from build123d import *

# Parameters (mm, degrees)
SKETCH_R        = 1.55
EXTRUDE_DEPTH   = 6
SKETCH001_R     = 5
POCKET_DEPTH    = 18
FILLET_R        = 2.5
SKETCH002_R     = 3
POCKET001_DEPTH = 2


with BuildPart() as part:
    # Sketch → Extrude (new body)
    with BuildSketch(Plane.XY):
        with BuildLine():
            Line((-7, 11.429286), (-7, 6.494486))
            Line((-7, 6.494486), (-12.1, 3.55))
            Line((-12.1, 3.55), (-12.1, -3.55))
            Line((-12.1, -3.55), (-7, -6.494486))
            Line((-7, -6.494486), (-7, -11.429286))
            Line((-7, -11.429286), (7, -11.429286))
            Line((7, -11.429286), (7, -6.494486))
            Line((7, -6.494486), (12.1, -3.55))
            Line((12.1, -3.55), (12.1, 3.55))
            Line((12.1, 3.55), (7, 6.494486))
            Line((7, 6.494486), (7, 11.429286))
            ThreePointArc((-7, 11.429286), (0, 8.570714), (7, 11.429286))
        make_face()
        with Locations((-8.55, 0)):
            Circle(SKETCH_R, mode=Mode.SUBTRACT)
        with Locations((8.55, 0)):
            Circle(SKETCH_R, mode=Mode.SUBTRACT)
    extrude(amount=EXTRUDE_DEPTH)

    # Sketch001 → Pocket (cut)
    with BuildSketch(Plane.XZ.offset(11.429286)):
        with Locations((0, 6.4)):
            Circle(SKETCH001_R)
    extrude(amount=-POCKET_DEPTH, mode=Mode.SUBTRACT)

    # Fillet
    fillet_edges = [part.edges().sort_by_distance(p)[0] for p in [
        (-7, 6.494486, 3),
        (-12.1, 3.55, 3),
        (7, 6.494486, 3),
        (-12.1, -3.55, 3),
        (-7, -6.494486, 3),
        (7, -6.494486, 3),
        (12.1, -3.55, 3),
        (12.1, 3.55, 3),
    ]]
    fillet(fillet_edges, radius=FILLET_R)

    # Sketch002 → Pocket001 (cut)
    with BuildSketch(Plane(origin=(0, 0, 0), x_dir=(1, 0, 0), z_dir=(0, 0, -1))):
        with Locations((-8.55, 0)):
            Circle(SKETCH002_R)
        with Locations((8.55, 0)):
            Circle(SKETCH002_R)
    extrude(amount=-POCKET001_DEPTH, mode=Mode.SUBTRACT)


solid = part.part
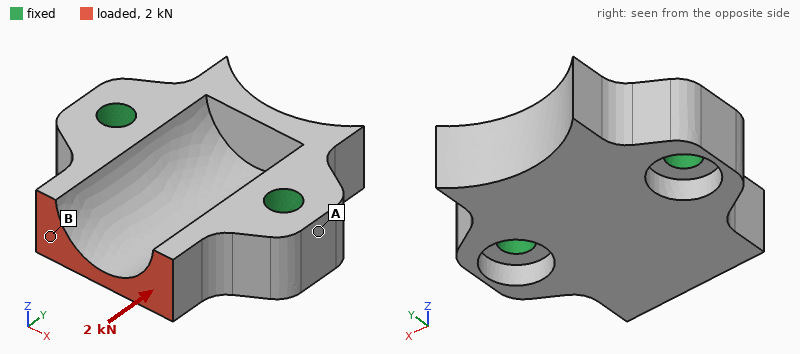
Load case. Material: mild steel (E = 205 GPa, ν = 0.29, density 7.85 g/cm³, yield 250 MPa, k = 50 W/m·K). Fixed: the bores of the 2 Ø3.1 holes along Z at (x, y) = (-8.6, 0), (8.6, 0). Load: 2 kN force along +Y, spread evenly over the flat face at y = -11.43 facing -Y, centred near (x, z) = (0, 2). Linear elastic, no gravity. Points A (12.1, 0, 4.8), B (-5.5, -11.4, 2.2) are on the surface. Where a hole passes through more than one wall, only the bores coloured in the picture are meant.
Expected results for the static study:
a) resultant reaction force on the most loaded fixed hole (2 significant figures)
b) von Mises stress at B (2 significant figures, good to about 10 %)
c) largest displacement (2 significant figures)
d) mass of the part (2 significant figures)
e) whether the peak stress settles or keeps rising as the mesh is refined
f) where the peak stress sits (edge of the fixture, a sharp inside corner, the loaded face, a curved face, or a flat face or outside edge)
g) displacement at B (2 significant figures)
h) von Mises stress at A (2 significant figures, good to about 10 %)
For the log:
1.0 kN
41 MPa
7.8 µm
12 g
keeps rising
edge of the fixture
5.3 µm
17 MPa
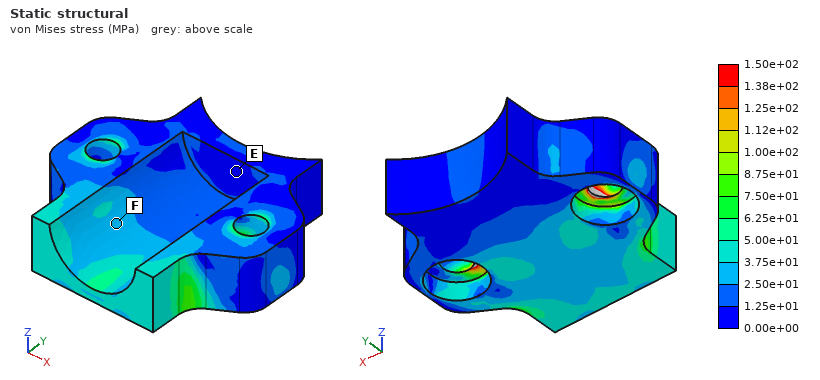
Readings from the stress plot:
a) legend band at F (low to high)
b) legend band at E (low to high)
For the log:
2.50e+01 to 3.75e+01 MPa
0.00e+00 to 1.25e+01 MPa
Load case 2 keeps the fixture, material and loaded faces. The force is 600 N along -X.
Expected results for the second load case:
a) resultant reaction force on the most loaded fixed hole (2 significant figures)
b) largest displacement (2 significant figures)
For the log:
440 N
6.7 µm
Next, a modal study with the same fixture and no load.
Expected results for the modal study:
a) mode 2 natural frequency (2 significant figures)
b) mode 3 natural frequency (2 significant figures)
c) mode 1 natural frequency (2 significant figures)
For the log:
36 kHz
37 kHz
26 kHz
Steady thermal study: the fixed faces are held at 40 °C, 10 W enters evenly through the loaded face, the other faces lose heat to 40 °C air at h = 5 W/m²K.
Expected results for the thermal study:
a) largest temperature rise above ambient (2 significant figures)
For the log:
41 K
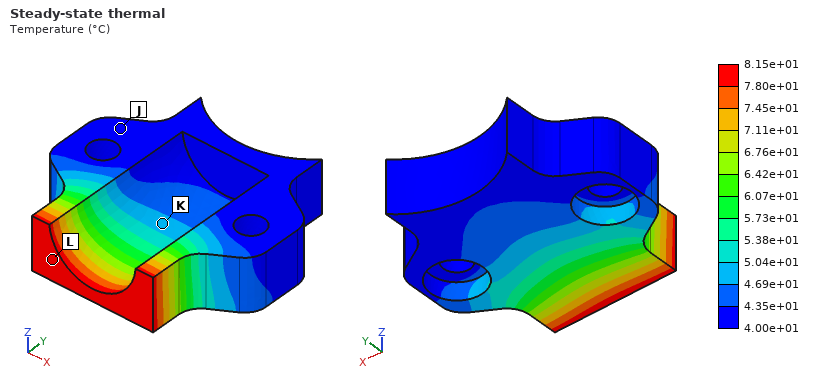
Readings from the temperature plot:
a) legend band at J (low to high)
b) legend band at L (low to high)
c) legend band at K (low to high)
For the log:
4.00e+01 to 4.35e+01 °C
7.80e+01 to 8.15e+01 °C
4.69e+01 to 5.04e+01 °C
